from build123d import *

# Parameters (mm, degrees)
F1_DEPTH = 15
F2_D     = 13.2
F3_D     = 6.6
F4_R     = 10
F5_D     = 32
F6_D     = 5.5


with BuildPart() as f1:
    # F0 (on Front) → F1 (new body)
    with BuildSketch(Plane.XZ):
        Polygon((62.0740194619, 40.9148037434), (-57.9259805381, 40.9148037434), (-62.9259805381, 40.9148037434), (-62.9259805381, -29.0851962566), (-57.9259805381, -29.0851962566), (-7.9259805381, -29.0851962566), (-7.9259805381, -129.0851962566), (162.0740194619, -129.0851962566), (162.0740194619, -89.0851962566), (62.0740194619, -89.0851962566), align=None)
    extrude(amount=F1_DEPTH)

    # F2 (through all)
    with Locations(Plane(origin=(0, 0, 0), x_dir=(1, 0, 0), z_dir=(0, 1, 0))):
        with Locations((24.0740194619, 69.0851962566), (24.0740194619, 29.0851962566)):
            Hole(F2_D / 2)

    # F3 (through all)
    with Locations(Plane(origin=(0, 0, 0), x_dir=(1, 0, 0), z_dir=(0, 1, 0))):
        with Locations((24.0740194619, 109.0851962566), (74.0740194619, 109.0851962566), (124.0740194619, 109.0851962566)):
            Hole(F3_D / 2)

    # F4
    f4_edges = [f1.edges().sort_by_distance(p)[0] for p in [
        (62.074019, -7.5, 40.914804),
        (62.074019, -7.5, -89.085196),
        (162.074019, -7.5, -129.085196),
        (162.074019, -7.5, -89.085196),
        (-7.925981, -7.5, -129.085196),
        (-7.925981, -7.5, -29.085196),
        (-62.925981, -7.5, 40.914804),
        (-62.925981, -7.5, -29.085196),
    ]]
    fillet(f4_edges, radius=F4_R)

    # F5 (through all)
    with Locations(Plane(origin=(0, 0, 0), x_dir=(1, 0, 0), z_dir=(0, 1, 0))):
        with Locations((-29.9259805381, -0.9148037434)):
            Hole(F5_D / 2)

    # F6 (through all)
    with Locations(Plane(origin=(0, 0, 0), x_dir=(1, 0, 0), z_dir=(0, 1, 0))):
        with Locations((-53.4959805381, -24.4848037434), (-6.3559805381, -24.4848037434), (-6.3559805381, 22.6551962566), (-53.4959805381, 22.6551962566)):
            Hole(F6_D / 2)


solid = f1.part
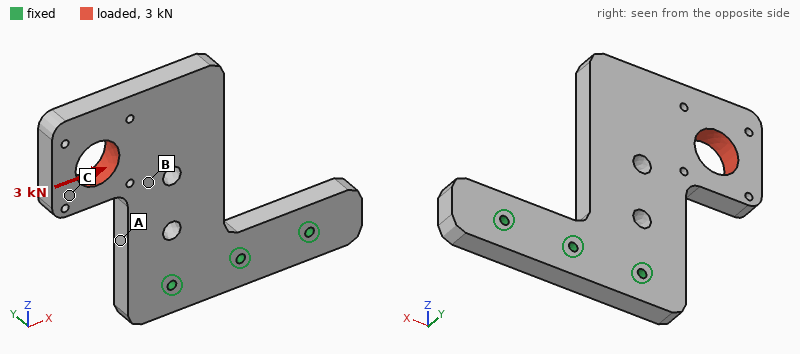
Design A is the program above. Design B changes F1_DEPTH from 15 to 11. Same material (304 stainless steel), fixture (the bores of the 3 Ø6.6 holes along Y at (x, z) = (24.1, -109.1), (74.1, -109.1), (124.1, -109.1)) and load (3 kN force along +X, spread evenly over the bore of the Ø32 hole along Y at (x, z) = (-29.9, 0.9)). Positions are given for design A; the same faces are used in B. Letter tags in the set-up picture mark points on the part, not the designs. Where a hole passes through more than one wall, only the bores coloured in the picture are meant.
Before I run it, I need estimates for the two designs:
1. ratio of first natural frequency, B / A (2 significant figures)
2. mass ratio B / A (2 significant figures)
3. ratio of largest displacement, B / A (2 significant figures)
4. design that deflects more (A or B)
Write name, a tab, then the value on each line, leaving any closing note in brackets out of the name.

ratio of first natural frequency, B / A	0.75
mass ratio B / A	0.73
ratio of largest displacement, B / A	1.4
design that deflects more	B
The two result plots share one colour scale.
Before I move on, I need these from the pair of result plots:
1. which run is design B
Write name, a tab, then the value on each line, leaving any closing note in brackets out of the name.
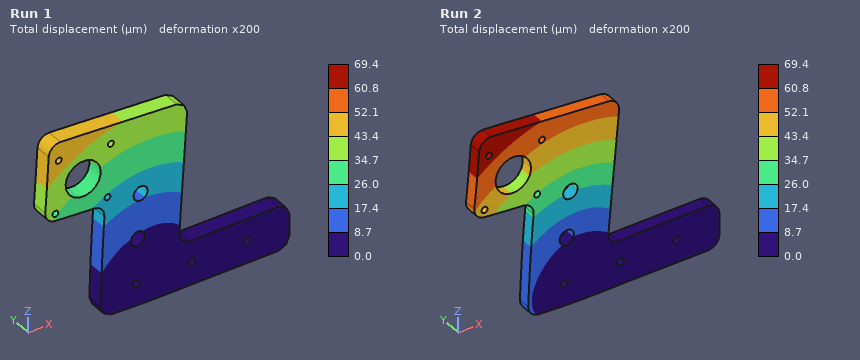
which run is design B	Run 2
